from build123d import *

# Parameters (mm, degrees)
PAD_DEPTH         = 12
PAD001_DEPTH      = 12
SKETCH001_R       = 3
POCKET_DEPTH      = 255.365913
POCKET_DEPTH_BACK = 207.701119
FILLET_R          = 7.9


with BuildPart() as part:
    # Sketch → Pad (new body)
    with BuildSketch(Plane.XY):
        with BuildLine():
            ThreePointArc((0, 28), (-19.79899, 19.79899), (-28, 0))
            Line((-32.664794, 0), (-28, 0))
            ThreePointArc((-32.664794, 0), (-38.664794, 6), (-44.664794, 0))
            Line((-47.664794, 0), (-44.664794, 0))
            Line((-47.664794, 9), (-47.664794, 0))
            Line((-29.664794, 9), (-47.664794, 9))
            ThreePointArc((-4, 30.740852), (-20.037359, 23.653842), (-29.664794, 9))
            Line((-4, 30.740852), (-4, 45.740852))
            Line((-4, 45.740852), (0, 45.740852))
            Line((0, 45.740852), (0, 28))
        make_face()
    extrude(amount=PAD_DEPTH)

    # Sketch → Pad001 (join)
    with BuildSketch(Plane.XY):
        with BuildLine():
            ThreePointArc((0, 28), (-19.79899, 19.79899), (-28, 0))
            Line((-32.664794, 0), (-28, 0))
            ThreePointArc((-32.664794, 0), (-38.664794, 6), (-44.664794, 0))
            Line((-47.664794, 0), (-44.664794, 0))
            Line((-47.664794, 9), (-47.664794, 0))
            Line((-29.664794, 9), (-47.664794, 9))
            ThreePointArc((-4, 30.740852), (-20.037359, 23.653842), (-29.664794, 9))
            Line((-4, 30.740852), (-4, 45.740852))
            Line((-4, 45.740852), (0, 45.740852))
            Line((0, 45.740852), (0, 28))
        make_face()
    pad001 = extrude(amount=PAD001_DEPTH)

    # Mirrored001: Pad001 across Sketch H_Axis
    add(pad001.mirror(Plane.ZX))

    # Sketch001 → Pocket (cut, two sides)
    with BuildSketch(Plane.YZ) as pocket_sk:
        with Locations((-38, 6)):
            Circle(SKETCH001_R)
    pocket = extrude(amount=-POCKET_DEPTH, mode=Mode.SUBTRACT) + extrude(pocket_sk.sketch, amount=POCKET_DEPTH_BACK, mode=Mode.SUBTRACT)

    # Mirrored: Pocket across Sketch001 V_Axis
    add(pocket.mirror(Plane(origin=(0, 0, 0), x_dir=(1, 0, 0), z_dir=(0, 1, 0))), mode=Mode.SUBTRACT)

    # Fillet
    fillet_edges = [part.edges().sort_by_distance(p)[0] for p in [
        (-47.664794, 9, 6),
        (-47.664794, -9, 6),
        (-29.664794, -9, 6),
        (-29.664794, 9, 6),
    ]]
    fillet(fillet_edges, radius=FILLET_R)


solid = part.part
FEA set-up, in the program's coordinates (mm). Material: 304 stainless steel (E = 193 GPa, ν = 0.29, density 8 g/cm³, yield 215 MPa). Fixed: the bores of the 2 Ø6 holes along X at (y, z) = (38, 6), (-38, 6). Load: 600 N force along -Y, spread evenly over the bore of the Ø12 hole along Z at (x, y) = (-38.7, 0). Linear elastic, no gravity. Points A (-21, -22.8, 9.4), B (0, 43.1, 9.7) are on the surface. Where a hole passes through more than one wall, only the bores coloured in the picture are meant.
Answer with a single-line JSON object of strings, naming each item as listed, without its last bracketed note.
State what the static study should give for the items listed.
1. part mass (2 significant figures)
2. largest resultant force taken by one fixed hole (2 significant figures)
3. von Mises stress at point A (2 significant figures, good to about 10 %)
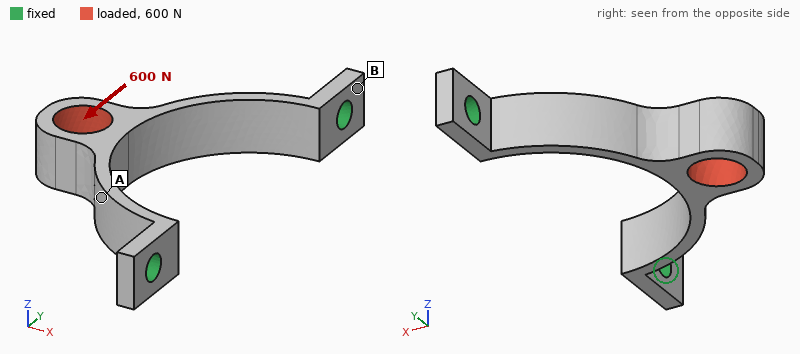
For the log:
{"part mass": "53 g", "largest resultant force taken by one fixed hole": "430 N", "von Mises stress at point A": "37 MPa"}
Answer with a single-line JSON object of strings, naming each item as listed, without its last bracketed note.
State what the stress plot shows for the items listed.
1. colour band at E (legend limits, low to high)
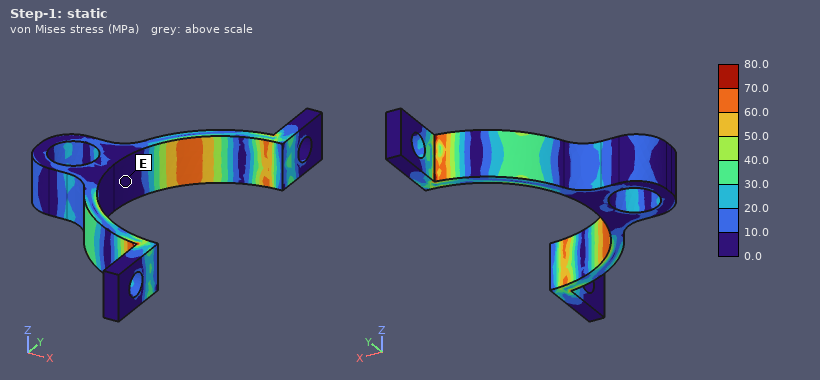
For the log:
{"colour band at E": "0.0 to 10.0 MPa"}
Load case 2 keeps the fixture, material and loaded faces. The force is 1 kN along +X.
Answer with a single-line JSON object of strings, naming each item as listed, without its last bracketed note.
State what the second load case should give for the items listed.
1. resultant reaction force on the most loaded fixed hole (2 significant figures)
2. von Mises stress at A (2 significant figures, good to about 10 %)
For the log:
{"resultant reaction force on the most loaded fixed hole": "630 N", "von Mises stress at A": "35 MPa"}
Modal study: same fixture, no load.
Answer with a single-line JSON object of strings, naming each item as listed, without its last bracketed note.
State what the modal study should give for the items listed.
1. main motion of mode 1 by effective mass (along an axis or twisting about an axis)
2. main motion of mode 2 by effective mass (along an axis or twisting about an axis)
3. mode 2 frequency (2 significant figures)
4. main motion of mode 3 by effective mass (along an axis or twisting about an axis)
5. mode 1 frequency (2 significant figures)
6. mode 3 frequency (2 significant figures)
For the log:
{"main motion of mode 1 by effective mass": "along Z", "main motion of mode 2 by effective mass": "along Y", "mode 2 frequency": "3100 Hz", "main motion of mode 3 by effective mass": "along X", "mode 1 frequency": "1600 Hz", "mode 3 frequency": "7000 Hz"}
